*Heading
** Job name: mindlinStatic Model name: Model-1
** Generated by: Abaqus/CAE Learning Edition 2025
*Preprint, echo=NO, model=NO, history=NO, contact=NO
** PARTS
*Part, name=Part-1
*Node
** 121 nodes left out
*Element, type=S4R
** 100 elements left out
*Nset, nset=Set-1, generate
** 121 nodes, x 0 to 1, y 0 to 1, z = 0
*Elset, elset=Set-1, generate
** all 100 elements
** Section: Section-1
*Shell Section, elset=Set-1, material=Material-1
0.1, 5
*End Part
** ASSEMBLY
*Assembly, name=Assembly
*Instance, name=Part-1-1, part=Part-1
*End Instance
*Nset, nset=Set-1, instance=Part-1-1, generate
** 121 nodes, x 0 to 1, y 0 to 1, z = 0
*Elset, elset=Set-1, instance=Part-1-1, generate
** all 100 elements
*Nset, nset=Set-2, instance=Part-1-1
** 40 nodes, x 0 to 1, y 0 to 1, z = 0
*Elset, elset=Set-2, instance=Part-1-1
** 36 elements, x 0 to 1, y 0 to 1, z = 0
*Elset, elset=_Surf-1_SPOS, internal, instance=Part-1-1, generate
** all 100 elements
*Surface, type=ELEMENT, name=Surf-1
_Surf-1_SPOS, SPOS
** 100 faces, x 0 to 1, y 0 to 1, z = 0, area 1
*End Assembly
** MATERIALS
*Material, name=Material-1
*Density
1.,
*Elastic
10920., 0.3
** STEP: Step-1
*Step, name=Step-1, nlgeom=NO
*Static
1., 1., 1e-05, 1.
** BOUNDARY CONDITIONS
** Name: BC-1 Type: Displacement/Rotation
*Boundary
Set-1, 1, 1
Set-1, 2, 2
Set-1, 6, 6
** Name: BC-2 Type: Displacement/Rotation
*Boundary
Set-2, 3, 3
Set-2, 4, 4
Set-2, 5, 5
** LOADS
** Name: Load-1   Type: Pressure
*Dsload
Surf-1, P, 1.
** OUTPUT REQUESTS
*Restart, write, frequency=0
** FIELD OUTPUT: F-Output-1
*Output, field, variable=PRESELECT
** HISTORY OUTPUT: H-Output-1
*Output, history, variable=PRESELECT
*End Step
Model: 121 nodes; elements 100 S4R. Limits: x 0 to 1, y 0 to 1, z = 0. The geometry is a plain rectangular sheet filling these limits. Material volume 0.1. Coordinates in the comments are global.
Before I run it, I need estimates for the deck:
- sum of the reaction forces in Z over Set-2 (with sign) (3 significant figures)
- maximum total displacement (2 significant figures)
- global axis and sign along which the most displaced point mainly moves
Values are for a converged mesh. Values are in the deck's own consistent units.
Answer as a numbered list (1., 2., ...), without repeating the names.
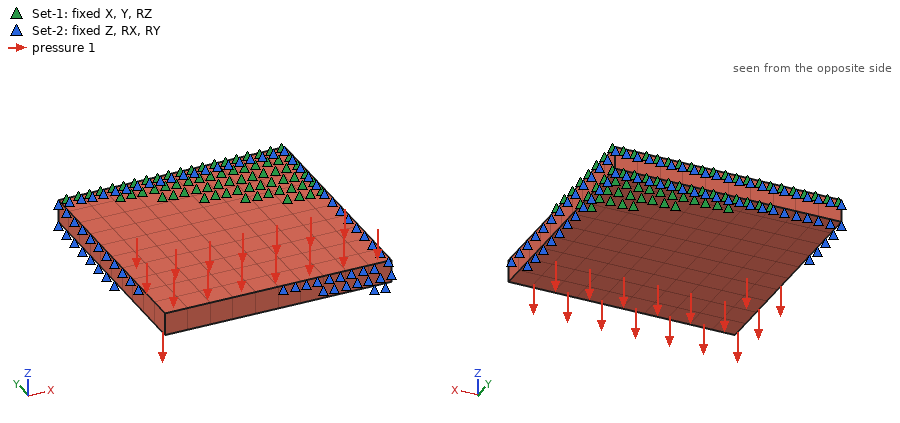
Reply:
1. 1.00
2. 0.0014
3. -Z
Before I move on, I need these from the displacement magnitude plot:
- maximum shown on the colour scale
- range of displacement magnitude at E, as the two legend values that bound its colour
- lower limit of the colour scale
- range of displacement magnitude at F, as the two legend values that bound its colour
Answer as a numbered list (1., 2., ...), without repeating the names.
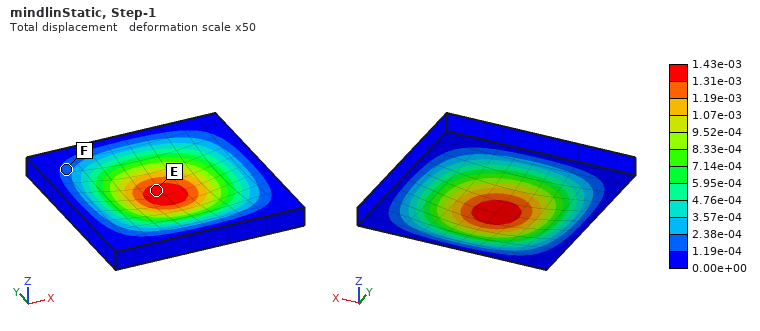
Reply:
1. 1.43e-03
2. 1.31e-03 to 1.43e-03
3. 0.00e+00
4. 1.19e-04 to 2.38e-04
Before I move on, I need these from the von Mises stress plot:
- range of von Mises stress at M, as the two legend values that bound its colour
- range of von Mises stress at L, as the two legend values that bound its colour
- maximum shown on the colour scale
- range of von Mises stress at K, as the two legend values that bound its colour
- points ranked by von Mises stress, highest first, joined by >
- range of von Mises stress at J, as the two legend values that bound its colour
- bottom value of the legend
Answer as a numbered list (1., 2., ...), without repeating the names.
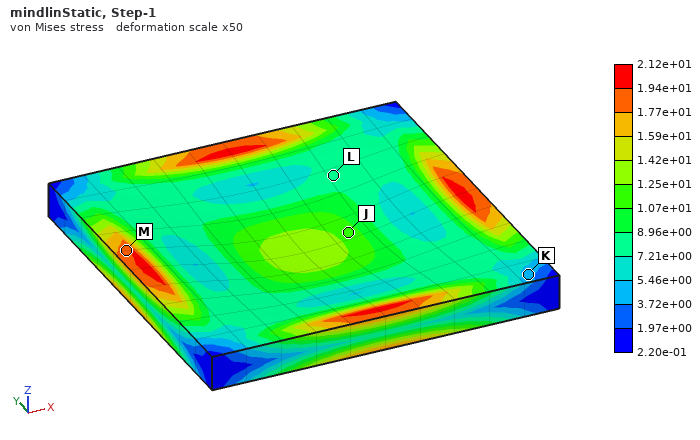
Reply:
1. 1.77e+01 to 1.94e+01
2. 7.21e+00 to 8.96e+00
3. 2.12e+01
4. 3.72e+00 to 5.46e+00
5. M > J > L > K
6. 1.07e+01 to 1.25e+01
7. 2.20e-01
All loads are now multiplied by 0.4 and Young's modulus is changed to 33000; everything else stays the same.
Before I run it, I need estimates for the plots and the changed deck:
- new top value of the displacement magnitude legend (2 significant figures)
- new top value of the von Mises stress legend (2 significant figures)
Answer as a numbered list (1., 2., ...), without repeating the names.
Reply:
1. 1.9e-04
2. 8.5
